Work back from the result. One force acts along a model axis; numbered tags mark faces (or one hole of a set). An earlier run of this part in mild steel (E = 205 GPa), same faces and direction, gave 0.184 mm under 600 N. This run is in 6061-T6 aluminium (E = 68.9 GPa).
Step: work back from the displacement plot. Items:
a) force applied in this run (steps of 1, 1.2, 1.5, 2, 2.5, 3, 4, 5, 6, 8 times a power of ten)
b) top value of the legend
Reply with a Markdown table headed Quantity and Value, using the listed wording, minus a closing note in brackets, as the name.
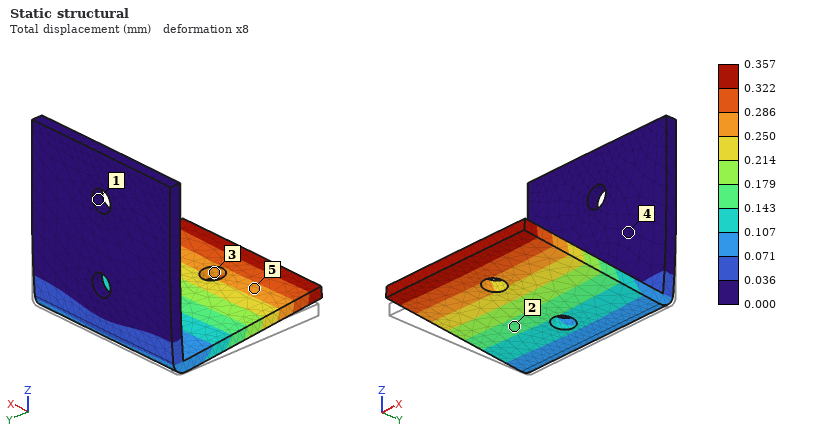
| Quantity | Value |
|---|---|
| force applied in this run | 400 N |
| top value of the legend | 0.357 mm |
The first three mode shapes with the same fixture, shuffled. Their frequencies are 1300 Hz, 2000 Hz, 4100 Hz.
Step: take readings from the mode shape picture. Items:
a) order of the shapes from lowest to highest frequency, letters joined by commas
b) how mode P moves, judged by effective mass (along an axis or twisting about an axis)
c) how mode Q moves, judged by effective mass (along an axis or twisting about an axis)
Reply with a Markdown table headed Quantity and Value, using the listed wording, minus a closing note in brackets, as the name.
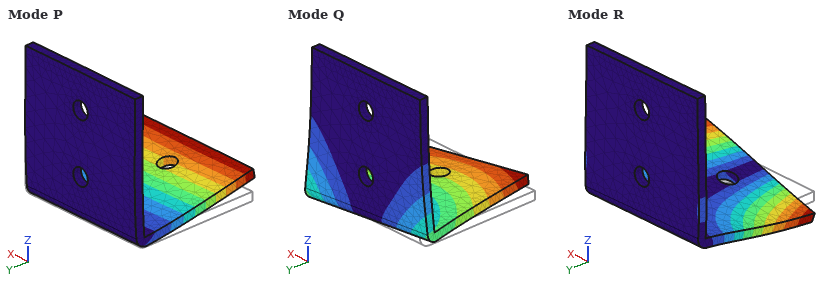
| Quantity | Value |
|---|---|
| order of the shapes from lowest to highest frequency, letters joined by commas | P, Q, R |
| how mode P moves, judged by effective mass | along Z |
| how mode Q moves, judged by effective mass | along X |
